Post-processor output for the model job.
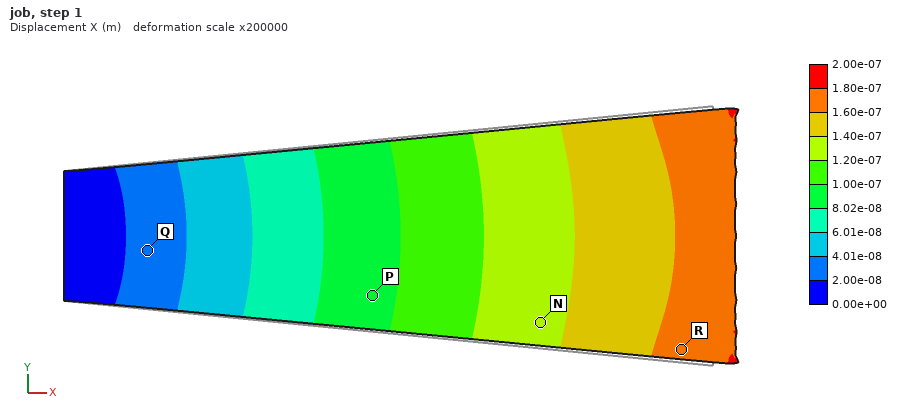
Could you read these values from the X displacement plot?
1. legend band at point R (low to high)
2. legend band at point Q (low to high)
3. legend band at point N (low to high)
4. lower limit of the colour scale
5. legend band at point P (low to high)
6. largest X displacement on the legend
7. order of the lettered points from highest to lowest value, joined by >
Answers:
1.60e-07 to 1.80e-07 m
2.00e-08 to 4.01e-08 m
1.20e-07 to 1.40e-07 m
0.00e+00 m
8.02e-08 to 1.00e-07 m
2.00e-07 m
R > N > P > Q
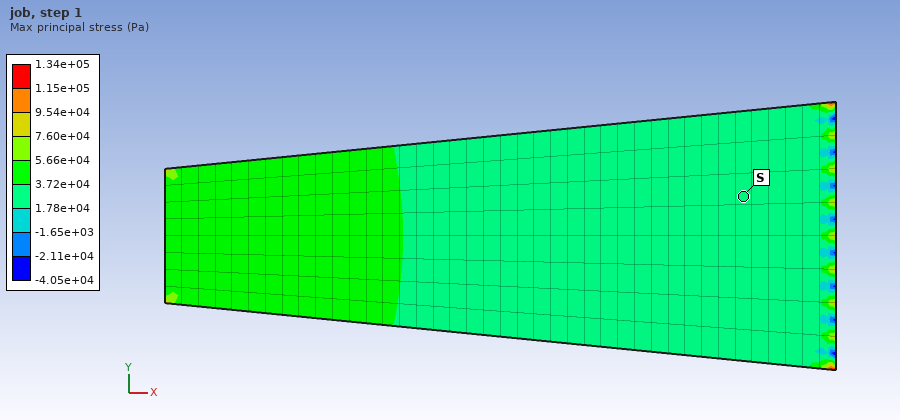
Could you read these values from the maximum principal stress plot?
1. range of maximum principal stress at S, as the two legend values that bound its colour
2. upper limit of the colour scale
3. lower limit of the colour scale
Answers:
1.78e+04 to 3.72e+04 Pa
1.34e+05 Pa
-4.05e+04 Pa
